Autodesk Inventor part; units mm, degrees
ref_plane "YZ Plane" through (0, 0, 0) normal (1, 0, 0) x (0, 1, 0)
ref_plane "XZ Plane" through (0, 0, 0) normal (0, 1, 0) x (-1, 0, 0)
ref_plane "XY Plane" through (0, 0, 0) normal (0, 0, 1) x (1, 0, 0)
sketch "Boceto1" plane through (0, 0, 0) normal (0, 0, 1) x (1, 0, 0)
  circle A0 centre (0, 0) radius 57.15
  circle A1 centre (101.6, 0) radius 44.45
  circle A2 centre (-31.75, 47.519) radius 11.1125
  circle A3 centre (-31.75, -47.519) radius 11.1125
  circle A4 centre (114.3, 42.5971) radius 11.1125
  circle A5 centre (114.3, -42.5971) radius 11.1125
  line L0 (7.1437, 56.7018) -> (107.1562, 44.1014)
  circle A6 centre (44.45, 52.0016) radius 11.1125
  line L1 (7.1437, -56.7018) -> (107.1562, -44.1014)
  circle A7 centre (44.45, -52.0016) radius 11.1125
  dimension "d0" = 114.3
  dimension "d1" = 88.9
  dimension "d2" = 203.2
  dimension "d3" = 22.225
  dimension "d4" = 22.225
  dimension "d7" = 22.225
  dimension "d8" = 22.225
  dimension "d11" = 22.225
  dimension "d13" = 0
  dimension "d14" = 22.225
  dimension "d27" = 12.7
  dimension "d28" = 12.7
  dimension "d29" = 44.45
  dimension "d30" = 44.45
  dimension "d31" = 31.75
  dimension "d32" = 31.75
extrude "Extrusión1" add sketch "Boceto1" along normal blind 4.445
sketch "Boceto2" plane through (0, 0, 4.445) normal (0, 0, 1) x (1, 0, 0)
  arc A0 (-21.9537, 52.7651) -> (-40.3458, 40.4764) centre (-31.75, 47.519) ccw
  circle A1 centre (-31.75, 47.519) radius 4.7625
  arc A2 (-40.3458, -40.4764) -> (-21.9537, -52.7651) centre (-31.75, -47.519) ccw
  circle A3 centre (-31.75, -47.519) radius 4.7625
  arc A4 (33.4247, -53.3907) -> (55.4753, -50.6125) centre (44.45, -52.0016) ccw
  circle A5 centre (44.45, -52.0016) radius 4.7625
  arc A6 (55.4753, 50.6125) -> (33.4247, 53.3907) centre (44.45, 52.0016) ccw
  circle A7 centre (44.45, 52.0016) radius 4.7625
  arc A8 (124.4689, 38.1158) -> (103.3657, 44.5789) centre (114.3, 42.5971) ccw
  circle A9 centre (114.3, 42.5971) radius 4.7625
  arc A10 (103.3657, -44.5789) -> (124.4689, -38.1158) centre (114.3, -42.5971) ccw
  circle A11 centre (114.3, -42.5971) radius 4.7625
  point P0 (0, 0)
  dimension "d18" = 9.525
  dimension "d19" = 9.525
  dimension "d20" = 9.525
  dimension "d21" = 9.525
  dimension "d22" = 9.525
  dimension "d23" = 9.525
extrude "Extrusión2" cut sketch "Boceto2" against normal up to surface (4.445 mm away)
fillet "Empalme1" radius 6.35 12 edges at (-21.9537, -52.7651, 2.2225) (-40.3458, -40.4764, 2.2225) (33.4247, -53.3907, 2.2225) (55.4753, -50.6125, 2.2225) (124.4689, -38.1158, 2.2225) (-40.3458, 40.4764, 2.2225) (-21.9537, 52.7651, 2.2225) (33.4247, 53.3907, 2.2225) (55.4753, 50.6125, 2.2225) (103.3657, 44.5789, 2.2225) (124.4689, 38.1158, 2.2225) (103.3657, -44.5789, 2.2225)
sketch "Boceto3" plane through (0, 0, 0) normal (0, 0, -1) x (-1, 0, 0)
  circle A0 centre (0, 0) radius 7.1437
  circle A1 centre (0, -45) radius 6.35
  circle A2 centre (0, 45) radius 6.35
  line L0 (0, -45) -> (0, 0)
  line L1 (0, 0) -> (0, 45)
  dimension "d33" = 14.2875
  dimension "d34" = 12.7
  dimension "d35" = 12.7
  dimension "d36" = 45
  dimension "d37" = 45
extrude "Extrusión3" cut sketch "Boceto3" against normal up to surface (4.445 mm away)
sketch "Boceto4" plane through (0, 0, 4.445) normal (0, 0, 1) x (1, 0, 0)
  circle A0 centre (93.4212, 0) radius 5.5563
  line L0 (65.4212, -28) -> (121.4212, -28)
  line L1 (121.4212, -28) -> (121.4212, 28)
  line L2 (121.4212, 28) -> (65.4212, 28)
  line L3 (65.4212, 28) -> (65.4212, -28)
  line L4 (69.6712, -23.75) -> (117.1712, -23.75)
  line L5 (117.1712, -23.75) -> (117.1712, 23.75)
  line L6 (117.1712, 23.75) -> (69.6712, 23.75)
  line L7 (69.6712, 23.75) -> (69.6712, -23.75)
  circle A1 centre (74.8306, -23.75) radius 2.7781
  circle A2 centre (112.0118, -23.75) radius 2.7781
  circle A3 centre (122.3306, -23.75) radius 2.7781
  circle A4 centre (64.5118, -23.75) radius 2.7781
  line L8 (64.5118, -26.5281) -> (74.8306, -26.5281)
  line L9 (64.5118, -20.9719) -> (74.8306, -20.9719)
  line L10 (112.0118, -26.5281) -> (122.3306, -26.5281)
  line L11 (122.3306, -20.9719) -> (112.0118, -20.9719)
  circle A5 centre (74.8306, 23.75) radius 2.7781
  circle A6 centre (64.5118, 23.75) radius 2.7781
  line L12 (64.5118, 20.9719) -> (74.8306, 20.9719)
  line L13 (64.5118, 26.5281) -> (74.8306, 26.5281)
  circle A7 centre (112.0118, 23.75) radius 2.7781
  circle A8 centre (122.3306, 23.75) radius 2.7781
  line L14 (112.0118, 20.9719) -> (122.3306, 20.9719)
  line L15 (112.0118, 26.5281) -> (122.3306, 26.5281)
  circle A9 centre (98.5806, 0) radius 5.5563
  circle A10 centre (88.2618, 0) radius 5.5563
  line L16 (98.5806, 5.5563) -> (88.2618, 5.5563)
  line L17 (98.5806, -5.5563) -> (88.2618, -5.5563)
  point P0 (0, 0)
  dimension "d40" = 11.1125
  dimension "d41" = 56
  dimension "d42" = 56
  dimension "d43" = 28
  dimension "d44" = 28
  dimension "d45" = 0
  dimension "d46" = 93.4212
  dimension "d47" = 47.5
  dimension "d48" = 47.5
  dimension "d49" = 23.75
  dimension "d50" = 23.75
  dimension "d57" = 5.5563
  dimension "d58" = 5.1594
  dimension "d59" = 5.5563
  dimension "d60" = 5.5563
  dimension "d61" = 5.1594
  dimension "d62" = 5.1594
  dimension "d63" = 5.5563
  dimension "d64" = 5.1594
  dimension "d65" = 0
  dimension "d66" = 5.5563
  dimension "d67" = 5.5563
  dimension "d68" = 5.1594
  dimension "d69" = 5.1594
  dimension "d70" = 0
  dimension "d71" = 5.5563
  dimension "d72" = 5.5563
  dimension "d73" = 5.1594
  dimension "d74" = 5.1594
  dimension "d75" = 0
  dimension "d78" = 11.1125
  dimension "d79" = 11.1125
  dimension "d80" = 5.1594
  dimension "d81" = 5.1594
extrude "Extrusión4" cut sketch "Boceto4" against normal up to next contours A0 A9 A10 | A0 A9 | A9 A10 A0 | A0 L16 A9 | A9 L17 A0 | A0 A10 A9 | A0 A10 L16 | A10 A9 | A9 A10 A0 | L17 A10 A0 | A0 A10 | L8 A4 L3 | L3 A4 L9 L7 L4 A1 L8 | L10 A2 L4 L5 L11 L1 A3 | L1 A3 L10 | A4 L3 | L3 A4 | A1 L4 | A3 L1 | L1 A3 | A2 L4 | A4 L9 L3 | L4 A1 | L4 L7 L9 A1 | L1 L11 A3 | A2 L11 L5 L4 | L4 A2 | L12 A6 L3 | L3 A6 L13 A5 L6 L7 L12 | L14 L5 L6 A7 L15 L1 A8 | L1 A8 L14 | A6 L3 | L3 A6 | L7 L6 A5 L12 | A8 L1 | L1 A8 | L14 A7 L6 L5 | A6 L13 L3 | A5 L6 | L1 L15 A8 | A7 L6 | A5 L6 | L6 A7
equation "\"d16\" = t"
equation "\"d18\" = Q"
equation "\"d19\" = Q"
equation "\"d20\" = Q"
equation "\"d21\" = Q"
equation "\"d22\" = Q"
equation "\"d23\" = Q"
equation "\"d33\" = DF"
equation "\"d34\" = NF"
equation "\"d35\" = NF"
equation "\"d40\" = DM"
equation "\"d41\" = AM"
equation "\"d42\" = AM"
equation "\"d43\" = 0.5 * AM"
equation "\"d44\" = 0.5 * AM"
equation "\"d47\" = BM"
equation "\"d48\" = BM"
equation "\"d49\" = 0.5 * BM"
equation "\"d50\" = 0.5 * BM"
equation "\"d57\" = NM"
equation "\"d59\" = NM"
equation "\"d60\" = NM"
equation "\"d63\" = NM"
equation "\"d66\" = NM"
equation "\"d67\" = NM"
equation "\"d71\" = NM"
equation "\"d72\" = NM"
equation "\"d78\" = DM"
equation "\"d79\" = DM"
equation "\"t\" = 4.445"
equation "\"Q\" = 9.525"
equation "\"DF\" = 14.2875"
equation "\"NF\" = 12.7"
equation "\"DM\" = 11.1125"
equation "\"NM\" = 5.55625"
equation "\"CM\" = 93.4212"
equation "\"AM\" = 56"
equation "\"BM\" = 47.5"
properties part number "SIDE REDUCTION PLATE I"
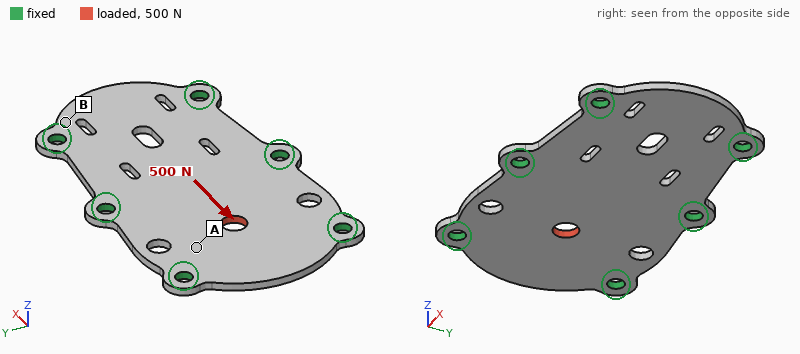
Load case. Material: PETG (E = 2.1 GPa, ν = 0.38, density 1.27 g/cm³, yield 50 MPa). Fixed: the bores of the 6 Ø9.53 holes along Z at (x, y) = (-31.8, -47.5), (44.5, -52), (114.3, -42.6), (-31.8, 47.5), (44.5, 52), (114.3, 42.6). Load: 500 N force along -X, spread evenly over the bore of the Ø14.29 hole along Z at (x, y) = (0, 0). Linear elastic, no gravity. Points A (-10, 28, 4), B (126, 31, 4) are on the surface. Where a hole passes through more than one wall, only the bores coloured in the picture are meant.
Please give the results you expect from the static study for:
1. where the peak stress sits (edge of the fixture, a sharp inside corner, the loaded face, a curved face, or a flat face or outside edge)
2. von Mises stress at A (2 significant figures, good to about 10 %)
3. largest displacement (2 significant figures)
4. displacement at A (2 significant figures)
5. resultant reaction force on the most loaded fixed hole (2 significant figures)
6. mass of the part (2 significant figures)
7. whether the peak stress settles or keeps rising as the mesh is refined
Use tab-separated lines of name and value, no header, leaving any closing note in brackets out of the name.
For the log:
where the peak stress sits	a sharp inside corner
von Mises stress at A	0.89 MPa
largest displacement	49 µm
displacement at A	18 µm
resultant reaction force on the most loaded fixed hole	120 N
mass of the part	100 g
whether the peak stress settles or keeps rising as the mesh is refined	keeps rising
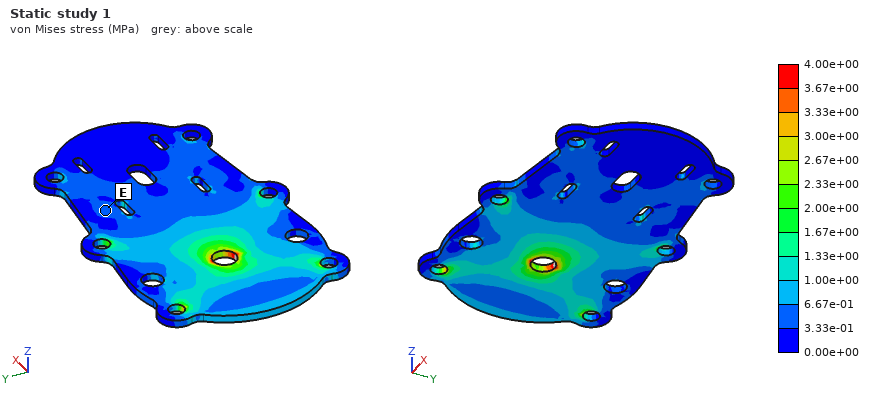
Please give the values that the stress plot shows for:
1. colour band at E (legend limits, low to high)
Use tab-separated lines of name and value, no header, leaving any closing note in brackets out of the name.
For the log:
colour band at E	3.33e-01 to 6.67e-01 MPa
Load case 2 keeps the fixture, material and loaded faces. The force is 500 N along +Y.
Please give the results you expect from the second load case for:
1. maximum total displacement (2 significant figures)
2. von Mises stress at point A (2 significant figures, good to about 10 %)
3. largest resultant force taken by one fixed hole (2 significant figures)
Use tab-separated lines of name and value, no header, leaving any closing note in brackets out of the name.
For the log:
maximum total displacement	42 µm
von Mises stress at point A	1.2 MPa
largest resultant force taken by one fixed hole	150 N
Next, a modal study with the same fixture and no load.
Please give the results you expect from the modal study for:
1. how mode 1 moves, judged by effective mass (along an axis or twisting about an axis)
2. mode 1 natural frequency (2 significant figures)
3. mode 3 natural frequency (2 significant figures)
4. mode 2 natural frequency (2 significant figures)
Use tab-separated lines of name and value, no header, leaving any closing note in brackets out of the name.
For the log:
how mode 1 moves, judged by effective mass	along Z
mode 1 natural frequency	540 Hz
mode 3 natural frequency	650 Hz
mode 2 natural frequency	630 Hz
